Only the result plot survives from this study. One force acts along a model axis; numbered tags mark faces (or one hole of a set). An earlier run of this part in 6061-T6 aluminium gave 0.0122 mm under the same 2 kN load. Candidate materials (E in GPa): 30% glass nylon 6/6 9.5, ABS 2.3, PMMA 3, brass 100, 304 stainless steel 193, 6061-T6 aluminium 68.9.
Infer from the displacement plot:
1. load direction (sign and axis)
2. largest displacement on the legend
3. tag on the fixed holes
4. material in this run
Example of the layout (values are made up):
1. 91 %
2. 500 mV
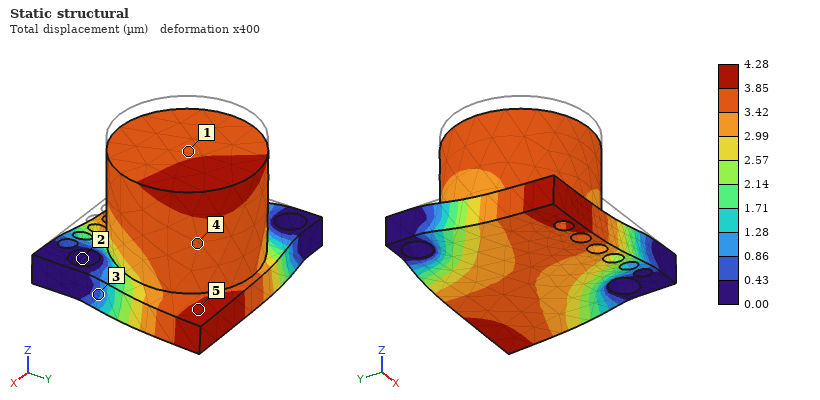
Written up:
1. -Z
2. 4.28 µm
3. 2
4. 304 stainless steel
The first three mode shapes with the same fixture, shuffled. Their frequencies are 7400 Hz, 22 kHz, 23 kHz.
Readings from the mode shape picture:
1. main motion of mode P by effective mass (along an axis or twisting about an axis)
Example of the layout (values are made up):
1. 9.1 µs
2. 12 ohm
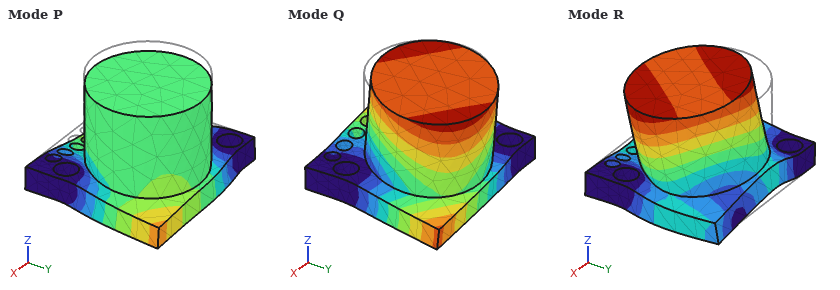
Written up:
1. along Z
